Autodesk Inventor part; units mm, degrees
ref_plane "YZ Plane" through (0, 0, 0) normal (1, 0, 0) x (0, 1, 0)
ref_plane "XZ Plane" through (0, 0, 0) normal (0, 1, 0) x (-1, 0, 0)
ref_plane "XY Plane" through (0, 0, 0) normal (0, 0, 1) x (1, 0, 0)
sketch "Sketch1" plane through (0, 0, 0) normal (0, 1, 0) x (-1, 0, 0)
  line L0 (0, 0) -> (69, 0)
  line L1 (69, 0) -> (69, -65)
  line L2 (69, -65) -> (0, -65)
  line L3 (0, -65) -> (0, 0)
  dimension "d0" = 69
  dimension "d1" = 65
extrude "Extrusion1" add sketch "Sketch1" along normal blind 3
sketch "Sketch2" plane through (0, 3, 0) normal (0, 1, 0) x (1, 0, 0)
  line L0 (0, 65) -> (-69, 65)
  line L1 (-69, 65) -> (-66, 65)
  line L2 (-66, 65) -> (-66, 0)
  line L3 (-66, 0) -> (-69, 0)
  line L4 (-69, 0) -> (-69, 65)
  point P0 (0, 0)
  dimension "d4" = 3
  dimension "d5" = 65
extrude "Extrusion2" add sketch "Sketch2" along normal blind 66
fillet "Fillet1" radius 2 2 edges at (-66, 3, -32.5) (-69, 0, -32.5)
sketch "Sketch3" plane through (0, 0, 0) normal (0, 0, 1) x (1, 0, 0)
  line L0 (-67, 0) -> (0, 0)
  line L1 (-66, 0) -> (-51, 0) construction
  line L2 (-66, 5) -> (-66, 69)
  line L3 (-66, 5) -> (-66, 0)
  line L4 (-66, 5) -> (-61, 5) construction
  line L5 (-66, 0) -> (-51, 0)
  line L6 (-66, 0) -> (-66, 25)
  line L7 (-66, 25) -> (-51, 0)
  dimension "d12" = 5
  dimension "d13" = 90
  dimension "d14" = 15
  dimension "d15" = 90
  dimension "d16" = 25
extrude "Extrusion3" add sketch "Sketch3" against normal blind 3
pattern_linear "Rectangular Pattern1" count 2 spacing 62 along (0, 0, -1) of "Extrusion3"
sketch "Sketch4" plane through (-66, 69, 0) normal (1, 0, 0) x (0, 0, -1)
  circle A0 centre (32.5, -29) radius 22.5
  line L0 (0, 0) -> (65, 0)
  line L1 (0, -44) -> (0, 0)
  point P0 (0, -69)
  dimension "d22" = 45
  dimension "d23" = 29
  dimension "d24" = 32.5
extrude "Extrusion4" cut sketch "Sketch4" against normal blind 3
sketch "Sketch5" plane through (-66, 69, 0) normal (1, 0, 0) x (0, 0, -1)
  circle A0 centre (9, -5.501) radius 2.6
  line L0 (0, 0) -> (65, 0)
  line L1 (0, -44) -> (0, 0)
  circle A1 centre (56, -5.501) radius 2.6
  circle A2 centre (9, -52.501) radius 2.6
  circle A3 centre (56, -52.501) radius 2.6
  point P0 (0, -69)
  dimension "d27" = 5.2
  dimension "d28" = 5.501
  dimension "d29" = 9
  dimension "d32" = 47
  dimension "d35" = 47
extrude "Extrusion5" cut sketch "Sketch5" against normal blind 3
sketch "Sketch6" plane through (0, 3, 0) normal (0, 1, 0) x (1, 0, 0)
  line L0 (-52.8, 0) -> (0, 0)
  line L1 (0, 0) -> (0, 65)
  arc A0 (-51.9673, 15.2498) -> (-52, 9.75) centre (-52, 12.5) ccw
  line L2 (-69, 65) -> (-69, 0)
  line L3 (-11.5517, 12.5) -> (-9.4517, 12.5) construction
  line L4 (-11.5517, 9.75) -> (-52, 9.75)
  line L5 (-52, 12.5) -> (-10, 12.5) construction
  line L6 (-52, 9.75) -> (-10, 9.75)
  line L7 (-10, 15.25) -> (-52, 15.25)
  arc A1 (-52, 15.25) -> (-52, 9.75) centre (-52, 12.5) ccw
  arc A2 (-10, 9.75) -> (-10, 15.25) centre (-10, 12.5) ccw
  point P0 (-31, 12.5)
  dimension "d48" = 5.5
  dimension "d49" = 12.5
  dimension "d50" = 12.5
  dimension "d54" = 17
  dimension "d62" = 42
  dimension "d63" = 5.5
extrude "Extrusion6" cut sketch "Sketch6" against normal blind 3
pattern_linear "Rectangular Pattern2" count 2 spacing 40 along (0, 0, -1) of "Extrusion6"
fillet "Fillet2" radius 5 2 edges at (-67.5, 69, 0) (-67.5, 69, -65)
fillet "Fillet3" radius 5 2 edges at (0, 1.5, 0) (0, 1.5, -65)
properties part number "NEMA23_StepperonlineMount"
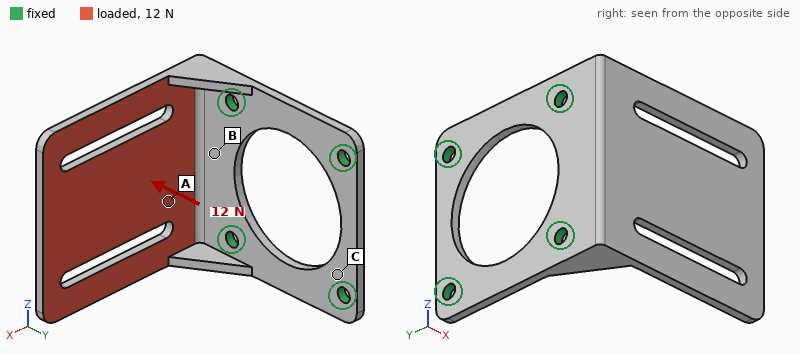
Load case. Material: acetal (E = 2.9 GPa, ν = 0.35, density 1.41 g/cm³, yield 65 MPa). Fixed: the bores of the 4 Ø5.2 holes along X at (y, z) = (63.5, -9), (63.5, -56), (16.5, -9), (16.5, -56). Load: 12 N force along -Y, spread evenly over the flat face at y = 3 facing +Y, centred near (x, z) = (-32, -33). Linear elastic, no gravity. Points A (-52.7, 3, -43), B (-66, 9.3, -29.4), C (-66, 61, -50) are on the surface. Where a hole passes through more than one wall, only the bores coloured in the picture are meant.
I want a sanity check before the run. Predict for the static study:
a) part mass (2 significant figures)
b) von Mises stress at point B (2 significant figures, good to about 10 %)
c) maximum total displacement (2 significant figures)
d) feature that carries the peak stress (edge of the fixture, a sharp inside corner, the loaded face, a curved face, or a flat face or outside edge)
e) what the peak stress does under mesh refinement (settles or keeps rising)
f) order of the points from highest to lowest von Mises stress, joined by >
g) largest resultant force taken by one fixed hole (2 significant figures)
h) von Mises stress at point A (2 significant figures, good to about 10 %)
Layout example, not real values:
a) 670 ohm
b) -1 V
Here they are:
a) 29 g
b) 1.4 MPa
c) 1.3 mm
d) edge of the fixture
e) keeps rising
f) A > B > C
g) 7.5 N
h) 2.5 MPa
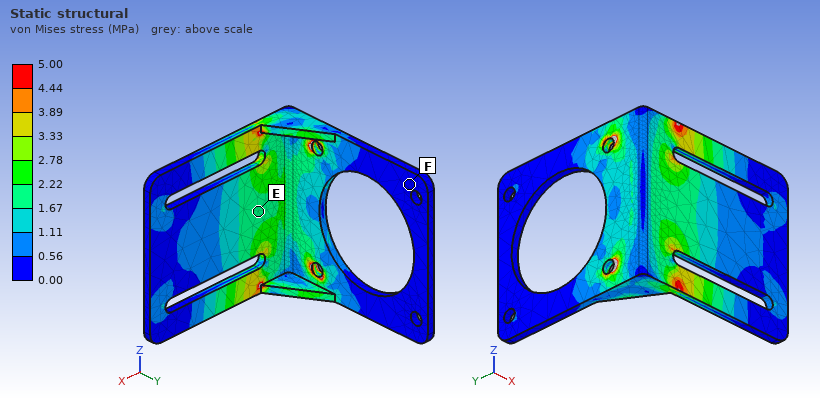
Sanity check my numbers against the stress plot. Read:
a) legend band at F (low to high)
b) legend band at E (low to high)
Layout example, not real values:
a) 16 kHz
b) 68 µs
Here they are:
a) 0.00 to 0.56 MPa
b) 1.67 to 2.22 MPa
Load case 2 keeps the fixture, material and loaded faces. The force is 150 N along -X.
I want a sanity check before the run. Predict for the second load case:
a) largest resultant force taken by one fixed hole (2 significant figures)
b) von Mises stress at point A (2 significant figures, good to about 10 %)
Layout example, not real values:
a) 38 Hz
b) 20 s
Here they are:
a) 78 N
b) 2.4 MPa
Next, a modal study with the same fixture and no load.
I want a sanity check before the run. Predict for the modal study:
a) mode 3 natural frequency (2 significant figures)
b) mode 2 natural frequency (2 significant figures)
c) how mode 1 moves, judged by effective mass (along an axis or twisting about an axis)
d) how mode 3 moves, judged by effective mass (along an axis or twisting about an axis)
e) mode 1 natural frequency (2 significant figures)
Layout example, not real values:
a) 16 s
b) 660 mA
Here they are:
a) 630 Hz
b) 400 Hz
c) along Y
d) along Z
e) 150 Hz
